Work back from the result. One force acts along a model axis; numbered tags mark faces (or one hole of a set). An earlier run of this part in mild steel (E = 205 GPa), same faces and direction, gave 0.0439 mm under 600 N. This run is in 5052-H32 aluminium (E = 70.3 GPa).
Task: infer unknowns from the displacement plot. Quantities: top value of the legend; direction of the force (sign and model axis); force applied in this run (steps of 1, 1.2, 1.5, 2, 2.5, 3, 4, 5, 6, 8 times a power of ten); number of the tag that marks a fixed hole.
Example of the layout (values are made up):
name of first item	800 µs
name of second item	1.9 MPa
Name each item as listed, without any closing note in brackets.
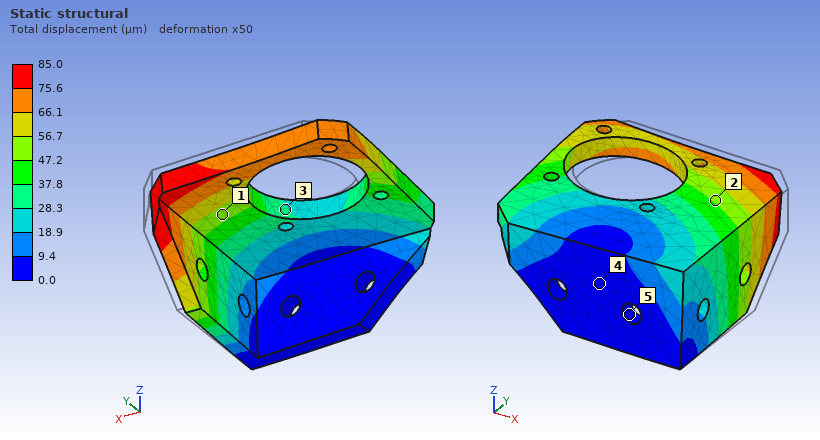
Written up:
top value of the legend	85.0 µm
direction of the force	-X
force applied in this run	400 N
number of the tag that marks a fixed hole	5
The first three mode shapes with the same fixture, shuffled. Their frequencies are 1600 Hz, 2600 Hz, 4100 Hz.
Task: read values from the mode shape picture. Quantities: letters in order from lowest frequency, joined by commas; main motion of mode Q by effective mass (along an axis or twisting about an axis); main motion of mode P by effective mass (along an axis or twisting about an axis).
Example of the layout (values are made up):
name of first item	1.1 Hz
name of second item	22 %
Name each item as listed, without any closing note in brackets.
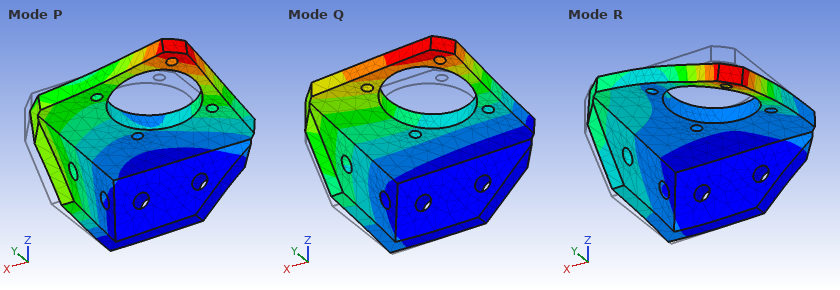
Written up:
letters in order from lowest frequency, joined by commas	Q, P, R
main motion of mode Q by effective mass	along Z
main motion of mode P by effective mass	along X
